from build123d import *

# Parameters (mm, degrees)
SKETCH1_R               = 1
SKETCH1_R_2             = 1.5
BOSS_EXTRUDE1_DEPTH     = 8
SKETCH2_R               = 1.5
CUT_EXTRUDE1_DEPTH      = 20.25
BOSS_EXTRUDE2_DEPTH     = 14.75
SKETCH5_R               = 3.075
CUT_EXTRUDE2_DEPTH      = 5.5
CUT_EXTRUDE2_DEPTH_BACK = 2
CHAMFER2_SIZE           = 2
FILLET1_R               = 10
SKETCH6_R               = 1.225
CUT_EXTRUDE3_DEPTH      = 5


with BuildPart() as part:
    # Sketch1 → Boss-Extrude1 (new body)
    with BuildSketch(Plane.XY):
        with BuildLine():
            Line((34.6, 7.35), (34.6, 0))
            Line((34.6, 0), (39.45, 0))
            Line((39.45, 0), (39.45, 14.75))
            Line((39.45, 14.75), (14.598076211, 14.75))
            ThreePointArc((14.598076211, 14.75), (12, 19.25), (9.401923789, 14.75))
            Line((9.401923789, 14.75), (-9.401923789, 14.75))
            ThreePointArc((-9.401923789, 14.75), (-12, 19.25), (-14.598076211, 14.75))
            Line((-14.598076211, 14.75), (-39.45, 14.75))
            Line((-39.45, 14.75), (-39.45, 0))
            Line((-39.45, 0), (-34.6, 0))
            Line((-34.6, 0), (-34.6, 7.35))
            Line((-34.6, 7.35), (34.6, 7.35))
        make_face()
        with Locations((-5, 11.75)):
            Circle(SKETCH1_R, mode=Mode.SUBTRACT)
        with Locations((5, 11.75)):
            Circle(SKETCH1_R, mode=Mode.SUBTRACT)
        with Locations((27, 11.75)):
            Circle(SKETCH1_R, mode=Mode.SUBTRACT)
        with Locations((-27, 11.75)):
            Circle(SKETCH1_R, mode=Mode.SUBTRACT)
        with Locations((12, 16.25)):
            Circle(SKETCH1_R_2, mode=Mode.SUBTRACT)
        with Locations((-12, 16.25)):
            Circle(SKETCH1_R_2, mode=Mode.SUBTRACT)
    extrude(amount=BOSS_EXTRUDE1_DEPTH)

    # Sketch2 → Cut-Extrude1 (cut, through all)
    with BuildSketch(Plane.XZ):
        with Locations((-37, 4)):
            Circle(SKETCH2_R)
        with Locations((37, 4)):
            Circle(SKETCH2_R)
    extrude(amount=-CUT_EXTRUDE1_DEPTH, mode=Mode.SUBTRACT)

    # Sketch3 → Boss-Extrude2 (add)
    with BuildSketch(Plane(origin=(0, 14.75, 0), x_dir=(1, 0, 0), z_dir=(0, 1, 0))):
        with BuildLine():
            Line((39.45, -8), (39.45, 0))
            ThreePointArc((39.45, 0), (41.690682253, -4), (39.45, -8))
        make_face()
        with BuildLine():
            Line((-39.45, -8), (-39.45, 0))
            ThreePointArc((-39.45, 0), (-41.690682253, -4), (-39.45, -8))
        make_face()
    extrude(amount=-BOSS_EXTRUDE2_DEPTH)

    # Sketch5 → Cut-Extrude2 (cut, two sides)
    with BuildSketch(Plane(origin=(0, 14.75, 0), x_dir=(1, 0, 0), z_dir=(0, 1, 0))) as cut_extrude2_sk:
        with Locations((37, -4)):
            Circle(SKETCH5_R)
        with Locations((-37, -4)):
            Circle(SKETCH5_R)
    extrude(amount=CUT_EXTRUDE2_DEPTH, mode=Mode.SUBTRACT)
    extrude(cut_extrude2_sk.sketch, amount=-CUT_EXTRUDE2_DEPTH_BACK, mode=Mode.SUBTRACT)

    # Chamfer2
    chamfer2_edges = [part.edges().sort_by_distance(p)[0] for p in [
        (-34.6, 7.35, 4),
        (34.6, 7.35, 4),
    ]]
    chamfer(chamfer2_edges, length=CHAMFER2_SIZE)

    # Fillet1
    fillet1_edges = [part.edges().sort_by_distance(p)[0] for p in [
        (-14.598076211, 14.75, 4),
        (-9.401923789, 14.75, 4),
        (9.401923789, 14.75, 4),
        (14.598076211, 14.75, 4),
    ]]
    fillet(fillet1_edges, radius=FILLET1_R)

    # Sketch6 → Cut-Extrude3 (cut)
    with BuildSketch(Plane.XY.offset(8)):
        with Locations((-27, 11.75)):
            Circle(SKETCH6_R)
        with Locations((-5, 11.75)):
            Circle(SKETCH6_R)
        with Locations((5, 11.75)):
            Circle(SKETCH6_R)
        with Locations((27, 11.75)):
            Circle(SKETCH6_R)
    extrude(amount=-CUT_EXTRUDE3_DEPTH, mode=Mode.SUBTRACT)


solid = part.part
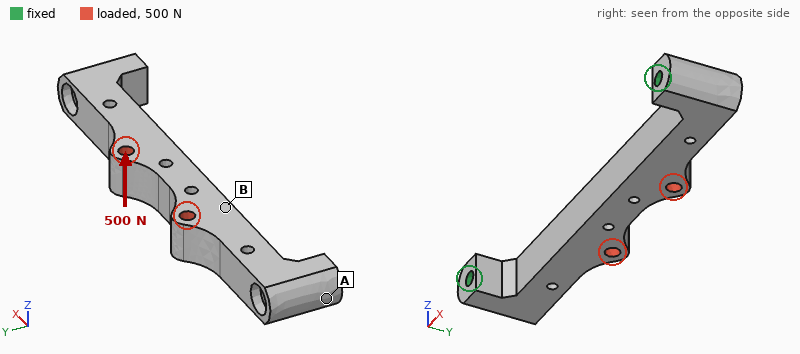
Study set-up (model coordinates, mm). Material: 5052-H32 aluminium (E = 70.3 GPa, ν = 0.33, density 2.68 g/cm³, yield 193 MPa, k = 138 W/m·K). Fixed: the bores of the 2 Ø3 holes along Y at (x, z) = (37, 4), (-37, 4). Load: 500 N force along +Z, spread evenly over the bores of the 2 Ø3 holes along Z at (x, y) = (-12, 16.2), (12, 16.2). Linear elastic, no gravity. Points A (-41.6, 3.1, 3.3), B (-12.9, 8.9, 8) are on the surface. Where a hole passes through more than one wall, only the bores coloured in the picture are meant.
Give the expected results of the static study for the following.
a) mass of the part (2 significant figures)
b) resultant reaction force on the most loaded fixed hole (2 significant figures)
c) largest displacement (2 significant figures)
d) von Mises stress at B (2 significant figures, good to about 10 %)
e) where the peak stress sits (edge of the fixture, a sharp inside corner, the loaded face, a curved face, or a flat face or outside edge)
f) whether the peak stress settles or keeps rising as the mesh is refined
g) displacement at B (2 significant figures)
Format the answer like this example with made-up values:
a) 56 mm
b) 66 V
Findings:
a) 15 g
b) 250 N
c) 62 µm
d) 24 MPa
e) edge of the fixture
f) keeps rising
g) 36 µm
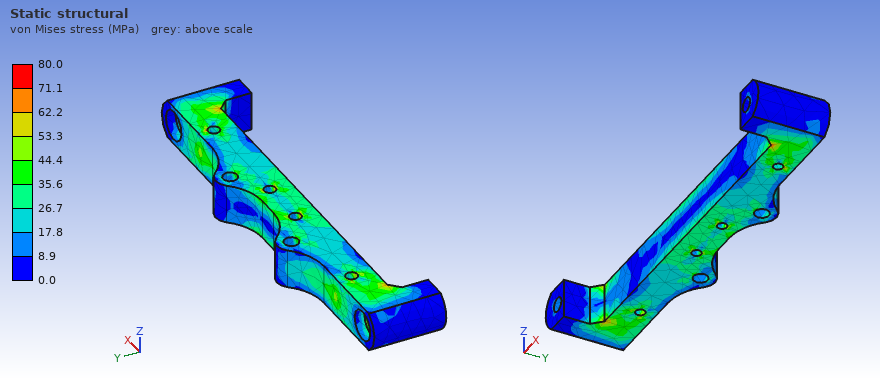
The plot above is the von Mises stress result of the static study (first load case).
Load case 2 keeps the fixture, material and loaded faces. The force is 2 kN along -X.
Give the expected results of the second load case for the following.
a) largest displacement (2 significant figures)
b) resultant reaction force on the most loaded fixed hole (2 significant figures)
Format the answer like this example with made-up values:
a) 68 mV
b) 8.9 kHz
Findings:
a) 10 µm
b) 1.0 kN
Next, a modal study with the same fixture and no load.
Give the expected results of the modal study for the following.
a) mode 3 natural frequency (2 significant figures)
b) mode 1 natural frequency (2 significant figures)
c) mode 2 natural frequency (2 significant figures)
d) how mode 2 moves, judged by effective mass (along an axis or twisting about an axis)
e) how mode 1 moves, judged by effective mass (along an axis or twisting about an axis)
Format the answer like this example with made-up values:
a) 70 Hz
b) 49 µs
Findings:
a) 16 kHz
b) 6100 Hz
c) 6500 Hz
d) along Y
e) along Z
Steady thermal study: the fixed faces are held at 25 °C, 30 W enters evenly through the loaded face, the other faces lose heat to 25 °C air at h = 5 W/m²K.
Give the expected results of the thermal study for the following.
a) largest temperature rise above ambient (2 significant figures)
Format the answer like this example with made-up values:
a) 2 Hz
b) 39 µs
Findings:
a) 51 K
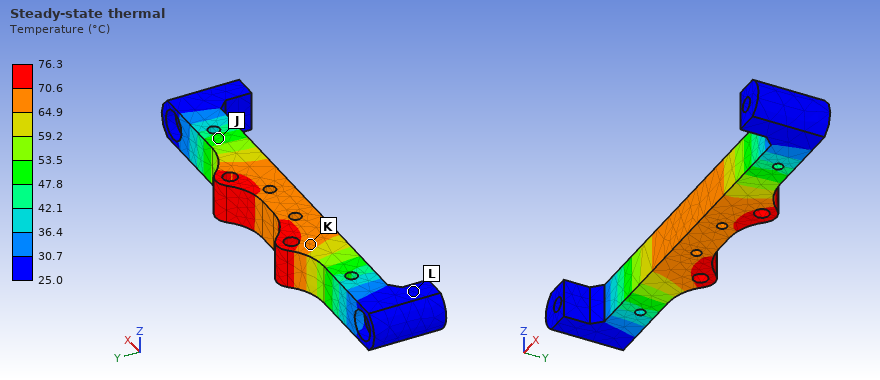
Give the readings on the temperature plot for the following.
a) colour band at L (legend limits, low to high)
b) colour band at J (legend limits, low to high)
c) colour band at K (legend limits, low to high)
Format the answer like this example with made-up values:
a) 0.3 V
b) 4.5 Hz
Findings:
a) 25.0 to 30.7 °C
b) 47.8 to 53.5 °C
c) 64.9 to 70.6 °C
